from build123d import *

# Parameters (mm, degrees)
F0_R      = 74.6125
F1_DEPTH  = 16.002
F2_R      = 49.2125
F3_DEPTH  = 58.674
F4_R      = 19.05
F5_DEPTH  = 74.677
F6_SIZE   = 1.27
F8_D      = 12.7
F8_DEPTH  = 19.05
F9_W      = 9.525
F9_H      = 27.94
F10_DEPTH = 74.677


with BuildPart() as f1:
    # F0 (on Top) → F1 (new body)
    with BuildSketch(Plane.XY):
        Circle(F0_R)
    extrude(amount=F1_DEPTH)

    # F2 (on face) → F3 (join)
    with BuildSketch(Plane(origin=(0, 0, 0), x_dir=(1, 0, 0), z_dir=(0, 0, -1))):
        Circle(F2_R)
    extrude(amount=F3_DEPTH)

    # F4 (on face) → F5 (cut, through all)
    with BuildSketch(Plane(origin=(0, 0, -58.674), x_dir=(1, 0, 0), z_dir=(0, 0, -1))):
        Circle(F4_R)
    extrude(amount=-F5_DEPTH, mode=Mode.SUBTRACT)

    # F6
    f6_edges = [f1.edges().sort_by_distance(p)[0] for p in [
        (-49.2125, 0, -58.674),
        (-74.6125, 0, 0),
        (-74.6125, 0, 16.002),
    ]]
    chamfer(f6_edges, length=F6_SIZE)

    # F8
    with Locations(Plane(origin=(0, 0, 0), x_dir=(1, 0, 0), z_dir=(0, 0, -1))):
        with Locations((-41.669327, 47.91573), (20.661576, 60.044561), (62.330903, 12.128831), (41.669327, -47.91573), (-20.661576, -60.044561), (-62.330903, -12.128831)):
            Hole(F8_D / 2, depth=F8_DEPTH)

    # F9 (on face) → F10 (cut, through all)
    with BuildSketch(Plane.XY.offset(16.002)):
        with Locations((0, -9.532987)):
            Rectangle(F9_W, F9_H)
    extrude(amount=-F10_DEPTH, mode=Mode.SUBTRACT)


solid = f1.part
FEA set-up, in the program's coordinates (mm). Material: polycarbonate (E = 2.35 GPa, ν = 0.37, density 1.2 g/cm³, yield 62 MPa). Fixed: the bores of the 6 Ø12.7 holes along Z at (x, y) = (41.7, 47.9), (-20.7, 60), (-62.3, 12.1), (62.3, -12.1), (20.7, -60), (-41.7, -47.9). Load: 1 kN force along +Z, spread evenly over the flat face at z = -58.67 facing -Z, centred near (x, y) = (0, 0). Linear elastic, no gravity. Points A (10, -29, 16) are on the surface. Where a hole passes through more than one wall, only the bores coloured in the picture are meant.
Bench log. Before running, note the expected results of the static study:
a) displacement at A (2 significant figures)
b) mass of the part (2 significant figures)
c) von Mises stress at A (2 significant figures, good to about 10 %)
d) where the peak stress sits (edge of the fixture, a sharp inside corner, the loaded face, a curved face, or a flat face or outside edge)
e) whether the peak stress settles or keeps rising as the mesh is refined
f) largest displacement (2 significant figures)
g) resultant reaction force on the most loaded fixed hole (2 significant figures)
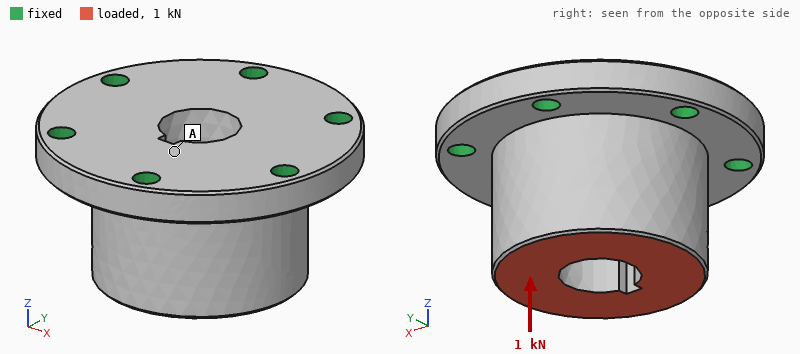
11 µm
750 g
0.16 MPa
edge of the fixture
keeps rising
13 µm
180 N
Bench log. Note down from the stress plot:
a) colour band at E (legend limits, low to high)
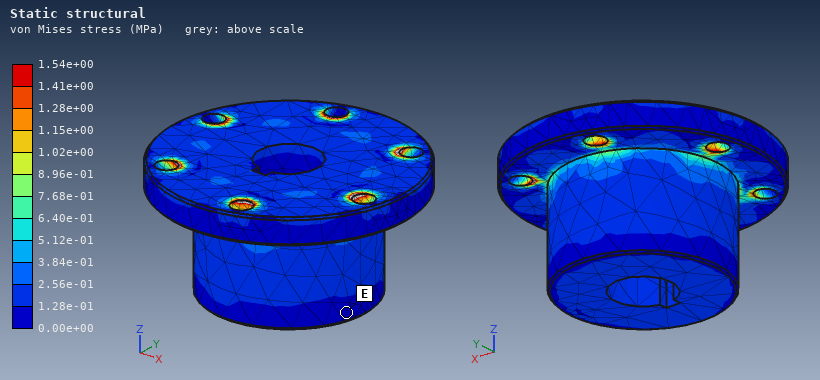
0.00e+00 to 1.28e-01 MPa
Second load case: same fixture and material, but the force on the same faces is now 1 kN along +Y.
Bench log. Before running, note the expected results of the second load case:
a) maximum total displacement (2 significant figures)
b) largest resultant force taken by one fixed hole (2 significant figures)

56 µm
440 N
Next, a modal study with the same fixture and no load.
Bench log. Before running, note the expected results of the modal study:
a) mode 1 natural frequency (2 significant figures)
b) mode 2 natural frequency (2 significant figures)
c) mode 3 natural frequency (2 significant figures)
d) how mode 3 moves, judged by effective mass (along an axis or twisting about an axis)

1600 Hz
1600 Hz
2000 Hz
along Z
